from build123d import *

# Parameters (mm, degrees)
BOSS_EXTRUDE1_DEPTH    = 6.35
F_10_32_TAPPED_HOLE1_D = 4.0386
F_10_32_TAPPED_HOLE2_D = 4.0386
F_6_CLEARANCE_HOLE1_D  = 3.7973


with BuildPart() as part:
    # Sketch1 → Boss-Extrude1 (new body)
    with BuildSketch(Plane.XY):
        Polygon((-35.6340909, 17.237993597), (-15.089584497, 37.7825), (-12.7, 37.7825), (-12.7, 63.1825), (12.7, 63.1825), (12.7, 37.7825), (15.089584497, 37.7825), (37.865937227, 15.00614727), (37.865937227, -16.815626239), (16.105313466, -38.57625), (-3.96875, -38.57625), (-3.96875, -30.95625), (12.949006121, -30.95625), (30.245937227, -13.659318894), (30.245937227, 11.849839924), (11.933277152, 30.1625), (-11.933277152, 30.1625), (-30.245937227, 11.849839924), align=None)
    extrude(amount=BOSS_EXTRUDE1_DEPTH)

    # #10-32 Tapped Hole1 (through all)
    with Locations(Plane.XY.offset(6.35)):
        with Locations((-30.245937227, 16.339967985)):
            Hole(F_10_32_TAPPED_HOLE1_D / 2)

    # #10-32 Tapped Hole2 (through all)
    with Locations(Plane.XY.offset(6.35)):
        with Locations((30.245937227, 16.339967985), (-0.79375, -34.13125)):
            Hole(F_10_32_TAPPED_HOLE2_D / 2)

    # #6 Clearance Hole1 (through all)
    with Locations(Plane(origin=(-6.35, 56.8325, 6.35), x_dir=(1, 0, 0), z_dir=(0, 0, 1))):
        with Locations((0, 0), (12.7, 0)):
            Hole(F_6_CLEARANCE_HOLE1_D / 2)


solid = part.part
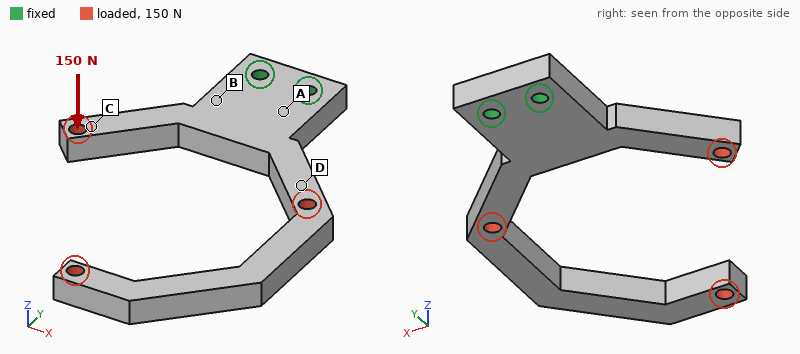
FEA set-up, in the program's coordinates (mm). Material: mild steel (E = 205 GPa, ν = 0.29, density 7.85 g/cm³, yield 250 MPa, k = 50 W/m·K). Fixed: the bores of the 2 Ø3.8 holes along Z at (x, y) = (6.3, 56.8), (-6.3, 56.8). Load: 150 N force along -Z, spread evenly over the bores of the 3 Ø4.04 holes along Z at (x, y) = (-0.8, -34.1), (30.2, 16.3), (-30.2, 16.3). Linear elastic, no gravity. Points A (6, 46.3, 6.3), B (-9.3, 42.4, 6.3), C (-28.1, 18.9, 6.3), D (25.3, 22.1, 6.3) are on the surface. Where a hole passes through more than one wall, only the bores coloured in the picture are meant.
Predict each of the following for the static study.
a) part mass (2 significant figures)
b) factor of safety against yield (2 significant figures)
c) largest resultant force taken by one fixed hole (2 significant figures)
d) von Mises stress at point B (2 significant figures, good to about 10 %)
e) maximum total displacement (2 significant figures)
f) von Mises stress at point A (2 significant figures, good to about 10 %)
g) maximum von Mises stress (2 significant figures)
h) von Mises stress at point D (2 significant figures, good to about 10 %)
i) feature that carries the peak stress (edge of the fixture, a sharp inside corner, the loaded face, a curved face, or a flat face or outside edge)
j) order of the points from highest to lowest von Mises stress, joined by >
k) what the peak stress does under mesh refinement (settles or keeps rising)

89 g
1.4
79 N
31 MPa
0.63 mm
42 MPa
180 MPa
85 MPa
the loaded face
D > A > B > C
settles
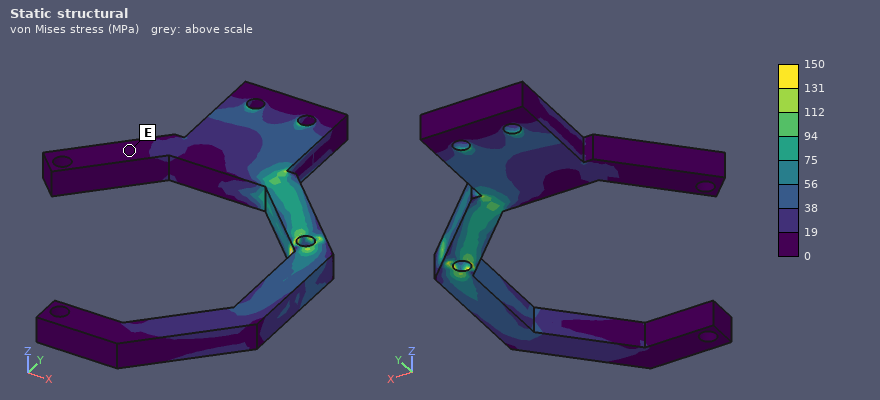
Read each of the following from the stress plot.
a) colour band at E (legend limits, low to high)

0 to 19 MPa
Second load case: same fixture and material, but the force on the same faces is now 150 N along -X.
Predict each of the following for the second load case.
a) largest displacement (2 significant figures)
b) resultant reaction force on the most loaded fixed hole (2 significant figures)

0.24 mm
570 N
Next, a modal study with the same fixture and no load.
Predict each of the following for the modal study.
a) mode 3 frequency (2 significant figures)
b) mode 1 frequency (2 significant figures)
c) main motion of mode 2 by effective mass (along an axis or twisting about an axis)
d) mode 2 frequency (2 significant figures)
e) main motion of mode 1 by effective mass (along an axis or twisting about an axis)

1500 Hz
440 Hz
along X
650 Hz
along Z
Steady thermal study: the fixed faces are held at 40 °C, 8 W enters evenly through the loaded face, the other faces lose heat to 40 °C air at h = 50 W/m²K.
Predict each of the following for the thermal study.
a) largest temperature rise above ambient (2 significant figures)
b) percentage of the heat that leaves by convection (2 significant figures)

50 K
66 %
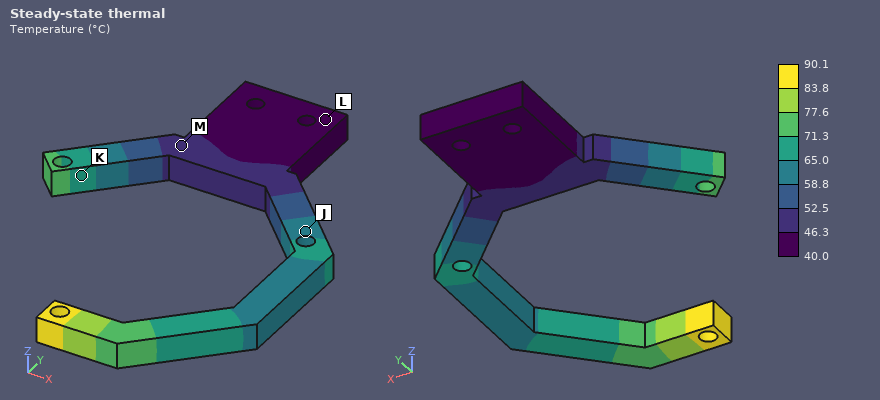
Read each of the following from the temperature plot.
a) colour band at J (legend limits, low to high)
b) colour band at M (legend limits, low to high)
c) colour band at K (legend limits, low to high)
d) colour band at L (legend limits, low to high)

58.8 to 65.0 °C
46.3 to 52.5 °C
65.0 to 71.3 °C
40.0 to 46.3 °C
